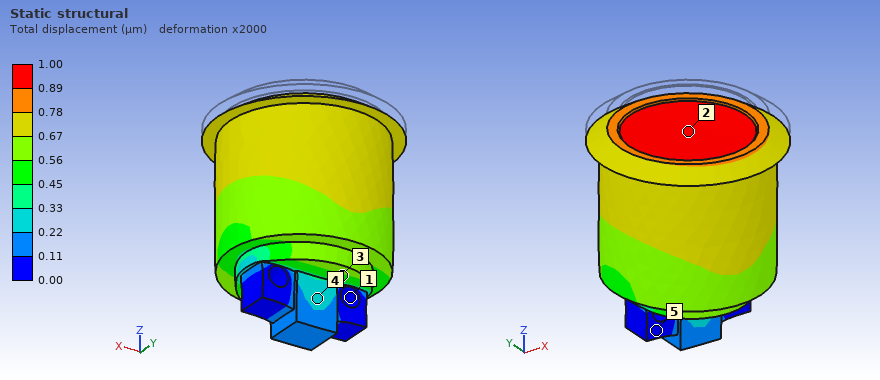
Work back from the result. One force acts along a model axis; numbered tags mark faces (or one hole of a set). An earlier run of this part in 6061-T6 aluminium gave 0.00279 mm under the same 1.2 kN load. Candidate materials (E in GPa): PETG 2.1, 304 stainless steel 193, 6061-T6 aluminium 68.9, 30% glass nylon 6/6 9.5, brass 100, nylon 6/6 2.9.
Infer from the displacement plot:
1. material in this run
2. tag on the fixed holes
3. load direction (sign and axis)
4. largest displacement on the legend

304 stainless steel
1
-Z
1.00 µm
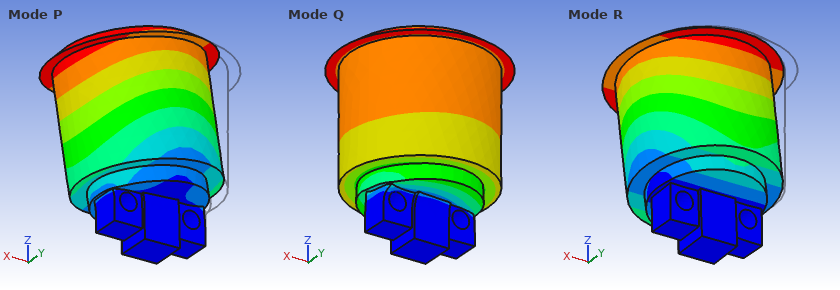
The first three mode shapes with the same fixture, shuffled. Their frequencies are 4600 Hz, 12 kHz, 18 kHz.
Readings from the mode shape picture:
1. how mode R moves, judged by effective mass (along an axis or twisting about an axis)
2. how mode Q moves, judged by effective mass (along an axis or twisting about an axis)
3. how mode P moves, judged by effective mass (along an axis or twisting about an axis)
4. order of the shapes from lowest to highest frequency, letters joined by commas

along Y
twisting about Z
along X
R, P, Q
